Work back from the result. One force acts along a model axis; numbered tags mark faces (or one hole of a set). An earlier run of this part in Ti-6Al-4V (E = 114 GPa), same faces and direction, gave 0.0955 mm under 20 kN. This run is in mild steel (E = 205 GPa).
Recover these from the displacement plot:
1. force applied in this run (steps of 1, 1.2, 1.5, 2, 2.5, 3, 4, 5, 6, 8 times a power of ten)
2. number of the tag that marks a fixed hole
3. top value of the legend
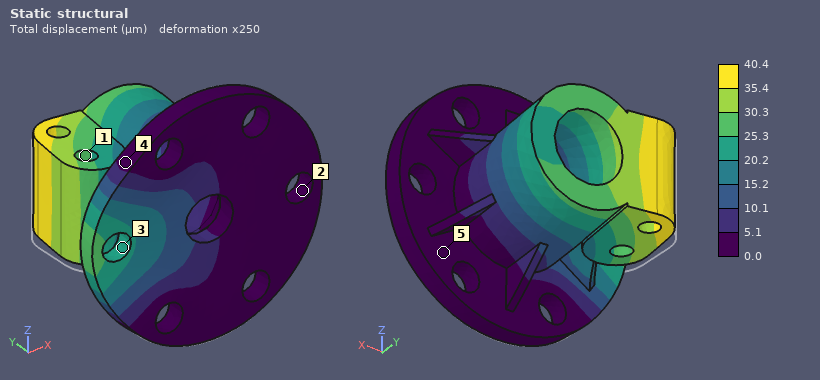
15 kN
2
40.4 µm
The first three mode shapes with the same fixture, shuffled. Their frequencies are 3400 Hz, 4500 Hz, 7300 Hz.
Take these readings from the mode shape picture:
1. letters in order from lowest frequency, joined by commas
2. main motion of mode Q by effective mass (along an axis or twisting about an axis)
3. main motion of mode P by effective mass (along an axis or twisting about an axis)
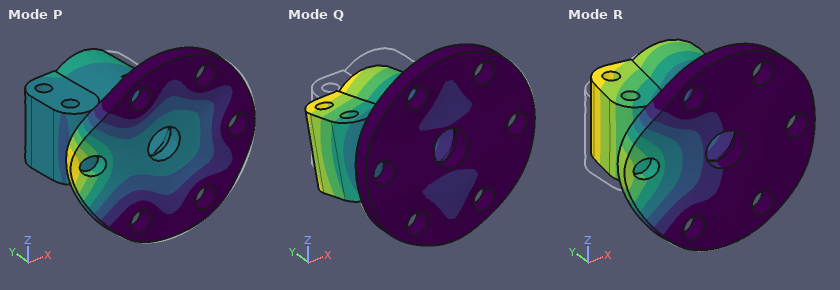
R, Q, P
along Z
along Y
